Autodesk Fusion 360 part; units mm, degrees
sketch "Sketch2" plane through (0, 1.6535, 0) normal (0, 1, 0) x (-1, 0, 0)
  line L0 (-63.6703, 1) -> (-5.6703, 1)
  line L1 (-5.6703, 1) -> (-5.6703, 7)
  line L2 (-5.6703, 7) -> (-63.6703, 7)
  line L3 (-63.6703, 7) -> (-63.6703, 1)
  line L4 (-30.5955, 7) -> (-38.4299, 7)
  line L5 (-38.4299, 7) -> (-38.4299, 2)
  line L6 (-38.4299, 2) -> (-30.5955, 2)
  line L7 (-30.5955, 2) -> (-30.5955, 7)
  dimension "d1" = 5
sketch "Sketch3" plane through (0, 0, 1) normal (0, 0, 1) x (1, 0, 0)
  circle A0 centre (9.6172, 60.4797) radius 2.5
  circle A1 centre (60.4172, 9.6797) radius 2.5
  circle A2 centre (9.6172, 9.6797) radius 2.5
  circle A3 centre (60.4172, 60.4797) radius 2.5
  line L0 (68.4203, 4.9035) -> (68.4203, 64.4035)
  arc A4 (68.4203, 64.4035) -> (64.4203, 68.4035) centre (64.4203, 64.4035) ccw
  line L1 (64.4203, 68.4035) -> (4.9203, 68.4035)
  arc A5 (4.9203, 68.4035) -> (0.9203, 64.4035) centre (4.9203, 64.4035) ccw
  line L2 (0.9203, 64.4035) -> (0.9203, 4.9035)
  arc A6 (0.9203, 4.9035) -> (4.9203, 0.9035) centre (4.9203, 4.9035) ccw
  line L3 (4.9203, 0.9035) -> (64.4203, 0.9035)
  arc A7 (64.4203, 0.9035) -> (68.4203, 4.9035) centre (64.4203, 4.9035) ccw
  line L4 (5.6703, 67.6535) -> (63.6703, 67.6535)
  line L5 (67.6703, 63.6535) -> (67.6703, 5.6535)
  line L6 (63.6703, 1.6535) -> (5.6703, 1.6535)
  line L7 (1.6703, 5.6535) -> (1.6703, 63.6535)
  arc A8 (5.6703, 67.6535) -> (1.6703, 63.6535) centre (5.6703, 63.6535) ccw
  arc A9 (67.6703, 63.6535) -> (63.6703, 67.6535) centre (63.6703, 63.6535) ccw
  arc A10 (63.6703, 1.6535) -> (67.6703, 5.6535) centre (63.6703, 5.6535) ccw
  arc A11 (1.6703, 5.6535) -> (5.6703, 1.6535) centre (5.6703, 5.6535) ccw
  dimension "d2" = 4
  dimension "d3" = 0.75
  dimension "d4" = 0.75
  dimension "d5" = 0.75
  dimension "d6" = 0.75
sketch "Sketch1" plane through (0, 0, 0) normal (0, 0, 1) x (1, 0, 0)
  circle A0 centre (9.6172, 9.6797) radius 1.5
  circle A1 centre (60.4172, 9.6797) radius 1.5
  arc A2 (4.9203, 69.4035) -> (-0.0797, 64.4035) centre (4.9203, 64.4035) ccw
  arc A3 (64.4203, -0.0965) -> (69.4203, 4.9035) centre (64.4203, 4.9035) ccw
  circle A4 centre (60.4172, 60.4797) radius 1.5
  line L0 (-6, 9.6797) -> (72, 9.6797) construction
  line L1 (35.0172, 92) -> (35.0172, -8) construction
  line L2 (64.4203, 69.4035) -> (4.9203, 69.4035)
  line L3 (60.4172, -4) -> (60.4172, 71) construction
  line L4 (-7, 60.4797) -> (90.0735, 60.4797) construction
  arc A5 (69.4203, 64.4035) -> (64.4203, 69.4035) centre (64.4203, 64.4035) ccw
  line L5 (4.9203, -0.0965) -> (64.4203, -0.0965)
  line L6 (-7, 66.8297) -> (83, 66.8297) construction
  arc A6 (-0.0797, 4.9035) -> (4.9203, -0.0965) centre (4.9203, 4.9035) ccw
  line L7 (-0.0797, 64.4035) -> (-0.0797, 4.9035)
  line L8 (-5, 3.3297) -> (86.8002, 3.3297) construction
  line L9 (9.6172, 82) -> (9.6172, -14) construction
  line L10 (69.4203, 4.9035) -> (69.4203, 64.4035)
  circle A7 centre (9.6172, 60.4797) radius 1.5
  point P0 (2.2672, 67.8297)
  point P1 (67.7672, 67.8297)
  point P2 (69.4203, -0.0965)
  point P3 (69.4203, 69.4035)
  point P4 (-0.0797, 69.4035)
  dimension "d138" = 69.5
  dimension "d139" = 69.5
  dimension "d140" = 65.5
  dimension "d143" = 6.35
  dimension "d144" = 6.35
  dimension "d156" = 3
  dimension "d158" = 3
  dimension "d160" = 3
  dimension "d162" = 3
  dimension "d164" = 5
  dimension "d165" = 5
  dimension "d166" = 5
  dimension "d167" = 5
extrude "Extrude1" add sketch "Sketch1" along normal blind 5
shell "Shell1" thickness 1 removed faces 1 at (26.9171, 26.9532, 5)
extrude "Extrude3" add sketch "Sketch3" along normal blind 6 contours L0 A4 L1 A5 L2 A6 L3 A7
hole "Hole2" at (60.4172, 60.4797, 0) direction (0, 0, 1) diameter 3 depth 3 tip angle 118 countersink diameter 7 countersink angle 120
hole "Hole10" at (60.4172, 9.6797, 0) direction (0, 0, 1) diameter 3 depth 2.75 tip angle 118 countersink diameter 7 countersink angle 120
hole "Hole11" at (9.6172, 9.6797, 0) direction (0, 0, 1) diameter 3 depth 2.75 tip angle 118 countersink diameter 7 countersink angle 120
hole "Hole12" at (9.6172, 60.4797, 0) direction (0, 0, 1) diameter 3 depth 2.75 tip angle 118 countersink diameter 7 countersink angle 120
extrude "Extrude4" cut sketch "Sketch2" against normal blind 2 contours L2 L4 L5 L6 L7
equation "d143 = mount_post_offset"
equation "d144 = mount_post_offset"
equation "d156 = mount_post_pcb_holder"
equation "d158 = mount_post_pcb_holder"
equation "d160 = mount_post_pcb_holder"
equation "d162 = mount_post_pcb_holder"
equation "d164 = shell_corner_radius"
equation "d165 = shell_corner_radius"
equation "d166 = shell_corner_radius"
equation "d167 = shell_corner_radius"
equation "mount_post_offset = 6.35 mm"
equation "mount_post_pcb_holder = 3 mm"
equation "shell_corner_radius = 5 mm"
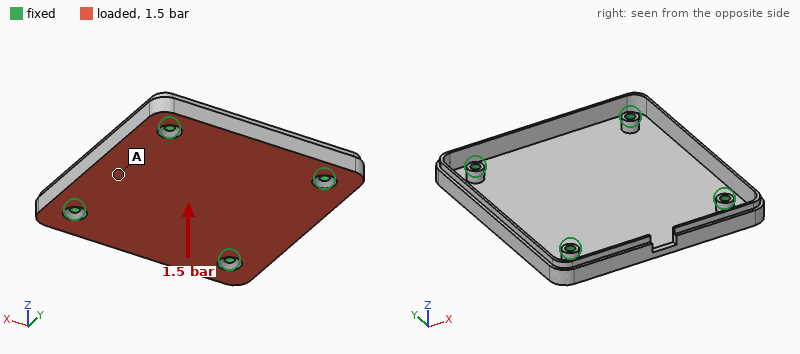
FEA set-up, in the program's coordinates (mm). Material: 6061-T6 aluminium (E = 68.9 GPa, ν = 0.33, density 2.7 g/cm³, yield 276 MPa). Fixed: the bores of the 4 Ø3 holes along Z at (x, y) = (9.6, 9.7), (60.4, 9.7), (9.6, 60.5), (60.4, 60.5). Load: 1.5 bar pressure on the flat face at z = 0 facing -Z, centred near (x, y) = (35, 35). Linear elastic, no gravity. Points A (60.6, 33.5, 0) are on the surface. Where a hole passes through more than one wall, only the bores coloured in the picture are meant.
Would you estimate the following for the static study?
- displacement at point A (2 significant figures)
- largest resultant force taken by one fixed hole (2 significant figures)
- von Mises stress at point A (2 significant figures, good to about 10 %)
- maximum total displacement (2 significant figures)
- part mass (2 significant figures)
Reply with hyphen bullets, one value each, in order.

- 0.25 mm
- 320 N
- 45 MPa
- 0.82 mm
- 19 g
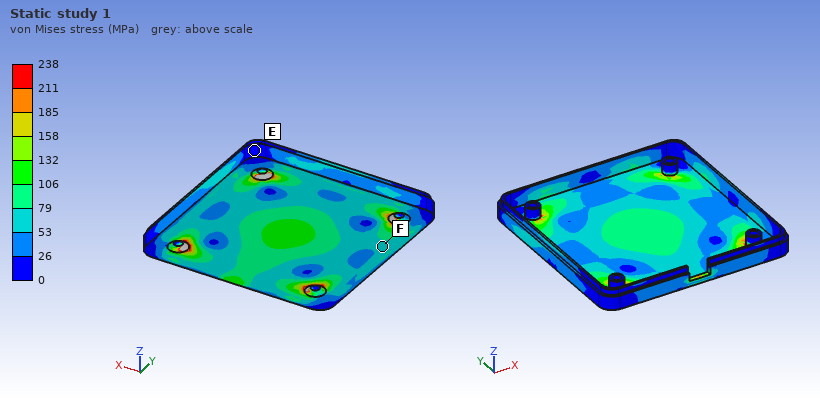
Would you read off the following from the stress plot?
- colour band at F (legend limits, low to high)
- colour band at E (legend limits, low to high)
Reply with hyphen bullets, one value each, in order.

- 53 to 79 MPa
- 0 to 26 MPa
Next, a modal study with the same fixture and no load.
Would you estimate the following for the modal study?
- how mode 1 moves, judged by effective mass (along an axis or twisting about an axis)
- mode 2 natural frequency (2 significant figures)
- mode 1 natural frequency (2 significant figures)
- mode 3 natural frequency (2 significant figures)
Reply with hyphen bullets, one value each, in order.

- along Z
- 2400 Hz
- 1600 Hz
- 3400 Hz
